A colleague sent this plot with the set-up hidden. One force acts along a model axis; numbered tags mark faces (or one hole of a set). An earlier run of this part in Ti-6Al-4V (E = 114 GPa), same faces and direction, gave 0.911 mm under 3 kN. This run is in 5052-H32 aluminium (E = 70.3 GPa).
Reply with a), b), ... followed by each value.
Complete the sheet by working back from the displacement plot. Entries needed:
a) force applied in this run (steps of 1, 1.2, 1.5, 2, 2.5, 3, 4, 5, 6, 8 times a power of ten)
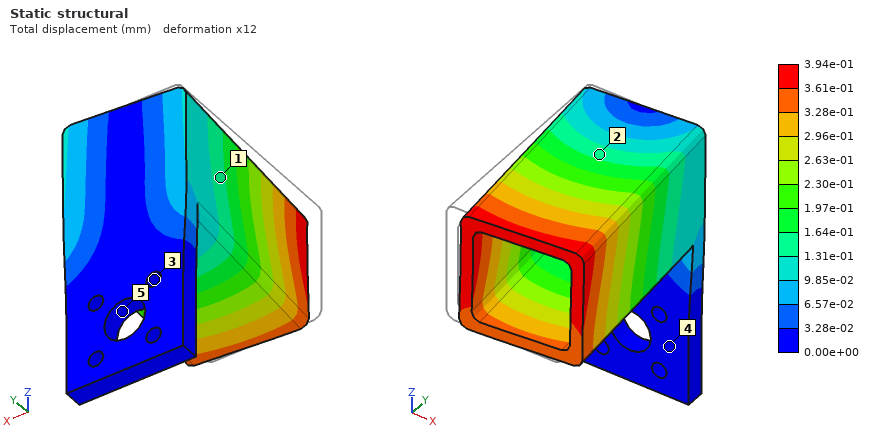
a) 800 N
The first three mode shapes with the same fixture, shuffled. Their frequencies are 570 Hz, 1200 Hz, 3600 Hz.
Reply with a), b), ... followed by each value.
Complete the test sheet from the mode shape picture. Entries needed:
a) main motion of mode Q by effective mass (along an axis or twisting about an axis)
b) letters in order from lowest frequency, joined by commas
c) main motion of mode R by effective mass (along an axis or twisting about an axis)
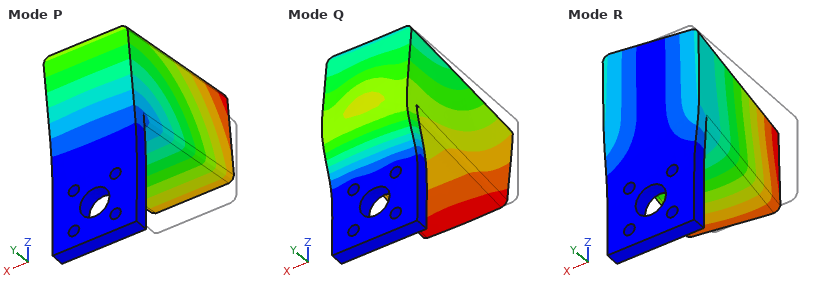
a) along Y
b) P, R, Q
c) along X
